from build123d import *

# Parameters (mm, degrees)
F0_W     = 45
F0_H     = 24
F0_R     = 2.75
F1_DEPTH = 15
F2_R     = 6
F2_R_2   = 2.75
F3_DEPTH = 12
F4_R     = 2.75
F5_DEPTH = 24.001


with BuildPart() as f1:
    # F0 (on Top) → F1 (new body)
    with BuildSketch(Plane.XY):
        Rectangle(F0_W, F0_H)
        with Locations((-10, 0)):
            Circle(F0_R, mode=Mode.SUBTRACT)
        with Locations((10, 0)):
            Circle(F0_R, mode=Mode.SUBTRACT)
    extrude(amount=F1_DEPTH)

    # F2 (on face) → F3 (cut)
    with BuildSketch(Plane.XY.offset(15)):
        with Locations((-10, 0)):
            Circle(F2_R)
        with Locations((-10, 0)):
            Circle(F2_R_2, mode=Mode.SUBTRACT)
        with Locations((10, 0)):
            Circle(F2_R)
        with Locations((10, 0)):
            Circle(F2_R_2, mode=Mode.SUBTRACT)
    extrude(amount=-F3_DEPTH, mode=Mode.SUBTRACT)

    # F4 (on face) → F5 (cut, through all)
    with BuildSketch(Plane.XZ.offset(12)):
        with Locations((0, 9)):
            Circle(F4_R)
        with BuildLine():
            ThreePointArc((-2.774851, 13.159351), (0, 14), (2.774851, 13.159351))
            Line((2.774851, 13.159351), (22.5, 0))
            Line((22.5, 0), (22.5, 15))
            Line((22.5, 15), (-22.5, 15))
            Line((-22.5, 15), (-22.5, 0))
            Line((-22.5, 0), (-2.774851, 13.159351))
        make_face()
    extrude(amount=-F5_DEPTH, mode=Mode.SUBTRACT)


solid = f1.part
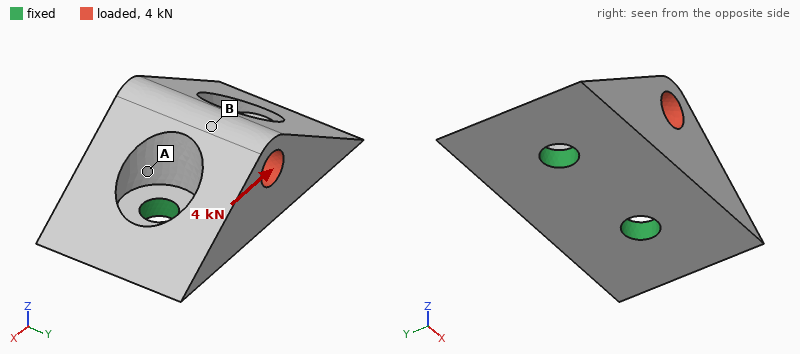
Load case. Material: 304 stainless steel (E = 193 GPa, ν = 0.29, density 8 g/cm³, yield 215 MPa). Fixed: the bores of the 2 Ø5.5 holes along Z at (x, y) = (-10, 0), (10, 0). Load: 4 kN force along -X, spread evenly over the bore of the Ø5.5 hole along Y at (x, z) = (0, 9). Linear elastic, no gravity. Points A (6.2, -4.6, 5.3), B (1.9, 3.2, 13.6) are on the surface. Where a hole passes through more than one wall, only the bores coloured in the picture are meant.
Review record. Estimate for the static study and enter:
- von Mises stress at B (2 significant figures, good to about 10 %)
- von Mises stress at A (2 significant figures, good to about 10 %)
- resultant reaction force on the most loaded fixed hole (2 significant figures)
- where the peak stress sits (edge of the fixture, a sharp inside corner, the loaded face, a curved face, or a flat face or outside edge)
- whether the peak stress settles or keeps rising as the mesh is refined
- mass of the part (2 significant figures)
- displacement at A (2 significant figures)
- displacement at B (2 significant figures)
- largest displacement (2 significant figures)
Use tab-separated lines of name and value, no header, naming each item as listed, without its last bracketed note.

von Mises stress at B	18 MPa
von Mises stress at A	40 MPa
resultant reaction force on the most loaded fixed hole	2.5 kN
where the peak stress sits	edge of the fixture
whether the peak stress settles or keeps rising as the mesh is refined	keeps rising
mass of the part	49 g
displacement at A	3.3 µm
displacement at B	7.3 µm
largest displacement	8.2 µm
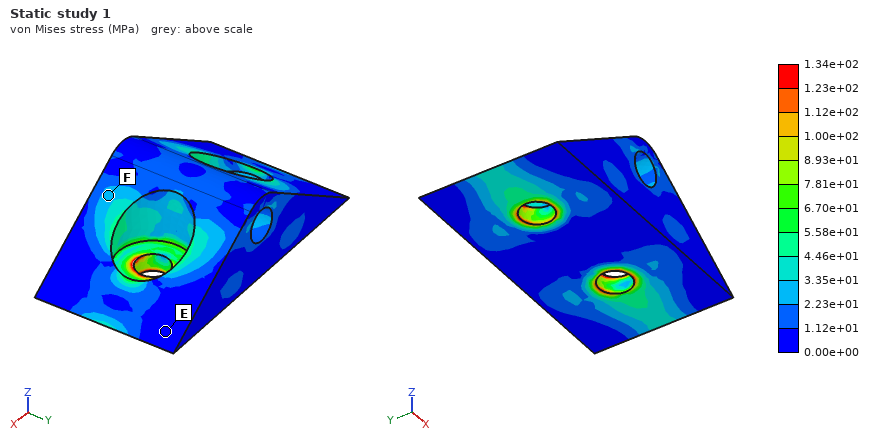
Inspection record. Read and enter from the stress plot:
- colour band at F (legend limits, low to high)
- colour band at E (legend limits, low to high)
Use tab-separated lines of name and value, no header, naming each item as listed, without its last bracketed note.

colour band at F	2.23e+01 to 3.35e+01 MPa
colour band at E	0.00e+00 to 1.12e+01 MPa
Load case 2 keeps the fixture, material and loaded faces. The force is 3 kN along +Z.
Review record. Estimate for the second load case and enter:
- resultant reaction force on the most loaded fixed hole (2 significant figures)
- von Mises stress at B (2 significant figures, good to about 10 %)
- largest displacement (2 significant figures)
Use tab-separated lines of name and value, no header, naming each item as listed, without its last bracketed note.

resultant reaction force on the most loaded fixed hole	1.6 kN
von Mises stress at B	15 MPa
largest displacement	4.7 µm
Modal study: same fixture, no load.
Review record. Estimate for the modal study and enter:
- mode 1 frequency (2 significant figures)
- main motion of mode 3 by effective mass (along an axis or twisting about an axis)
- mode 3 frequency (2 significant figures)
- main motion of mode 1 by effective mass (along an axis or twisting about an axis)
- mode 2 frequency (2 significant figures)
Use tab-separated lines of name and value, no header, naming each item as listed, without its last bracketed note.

mode 1 frequency	11 kHz
main motion of mode 3 by effective mass	along Z
mode 3 frequency	23 kHz
main motion of mode 1 by effective mass	along Y
mode 2 frequency	22 kHz
